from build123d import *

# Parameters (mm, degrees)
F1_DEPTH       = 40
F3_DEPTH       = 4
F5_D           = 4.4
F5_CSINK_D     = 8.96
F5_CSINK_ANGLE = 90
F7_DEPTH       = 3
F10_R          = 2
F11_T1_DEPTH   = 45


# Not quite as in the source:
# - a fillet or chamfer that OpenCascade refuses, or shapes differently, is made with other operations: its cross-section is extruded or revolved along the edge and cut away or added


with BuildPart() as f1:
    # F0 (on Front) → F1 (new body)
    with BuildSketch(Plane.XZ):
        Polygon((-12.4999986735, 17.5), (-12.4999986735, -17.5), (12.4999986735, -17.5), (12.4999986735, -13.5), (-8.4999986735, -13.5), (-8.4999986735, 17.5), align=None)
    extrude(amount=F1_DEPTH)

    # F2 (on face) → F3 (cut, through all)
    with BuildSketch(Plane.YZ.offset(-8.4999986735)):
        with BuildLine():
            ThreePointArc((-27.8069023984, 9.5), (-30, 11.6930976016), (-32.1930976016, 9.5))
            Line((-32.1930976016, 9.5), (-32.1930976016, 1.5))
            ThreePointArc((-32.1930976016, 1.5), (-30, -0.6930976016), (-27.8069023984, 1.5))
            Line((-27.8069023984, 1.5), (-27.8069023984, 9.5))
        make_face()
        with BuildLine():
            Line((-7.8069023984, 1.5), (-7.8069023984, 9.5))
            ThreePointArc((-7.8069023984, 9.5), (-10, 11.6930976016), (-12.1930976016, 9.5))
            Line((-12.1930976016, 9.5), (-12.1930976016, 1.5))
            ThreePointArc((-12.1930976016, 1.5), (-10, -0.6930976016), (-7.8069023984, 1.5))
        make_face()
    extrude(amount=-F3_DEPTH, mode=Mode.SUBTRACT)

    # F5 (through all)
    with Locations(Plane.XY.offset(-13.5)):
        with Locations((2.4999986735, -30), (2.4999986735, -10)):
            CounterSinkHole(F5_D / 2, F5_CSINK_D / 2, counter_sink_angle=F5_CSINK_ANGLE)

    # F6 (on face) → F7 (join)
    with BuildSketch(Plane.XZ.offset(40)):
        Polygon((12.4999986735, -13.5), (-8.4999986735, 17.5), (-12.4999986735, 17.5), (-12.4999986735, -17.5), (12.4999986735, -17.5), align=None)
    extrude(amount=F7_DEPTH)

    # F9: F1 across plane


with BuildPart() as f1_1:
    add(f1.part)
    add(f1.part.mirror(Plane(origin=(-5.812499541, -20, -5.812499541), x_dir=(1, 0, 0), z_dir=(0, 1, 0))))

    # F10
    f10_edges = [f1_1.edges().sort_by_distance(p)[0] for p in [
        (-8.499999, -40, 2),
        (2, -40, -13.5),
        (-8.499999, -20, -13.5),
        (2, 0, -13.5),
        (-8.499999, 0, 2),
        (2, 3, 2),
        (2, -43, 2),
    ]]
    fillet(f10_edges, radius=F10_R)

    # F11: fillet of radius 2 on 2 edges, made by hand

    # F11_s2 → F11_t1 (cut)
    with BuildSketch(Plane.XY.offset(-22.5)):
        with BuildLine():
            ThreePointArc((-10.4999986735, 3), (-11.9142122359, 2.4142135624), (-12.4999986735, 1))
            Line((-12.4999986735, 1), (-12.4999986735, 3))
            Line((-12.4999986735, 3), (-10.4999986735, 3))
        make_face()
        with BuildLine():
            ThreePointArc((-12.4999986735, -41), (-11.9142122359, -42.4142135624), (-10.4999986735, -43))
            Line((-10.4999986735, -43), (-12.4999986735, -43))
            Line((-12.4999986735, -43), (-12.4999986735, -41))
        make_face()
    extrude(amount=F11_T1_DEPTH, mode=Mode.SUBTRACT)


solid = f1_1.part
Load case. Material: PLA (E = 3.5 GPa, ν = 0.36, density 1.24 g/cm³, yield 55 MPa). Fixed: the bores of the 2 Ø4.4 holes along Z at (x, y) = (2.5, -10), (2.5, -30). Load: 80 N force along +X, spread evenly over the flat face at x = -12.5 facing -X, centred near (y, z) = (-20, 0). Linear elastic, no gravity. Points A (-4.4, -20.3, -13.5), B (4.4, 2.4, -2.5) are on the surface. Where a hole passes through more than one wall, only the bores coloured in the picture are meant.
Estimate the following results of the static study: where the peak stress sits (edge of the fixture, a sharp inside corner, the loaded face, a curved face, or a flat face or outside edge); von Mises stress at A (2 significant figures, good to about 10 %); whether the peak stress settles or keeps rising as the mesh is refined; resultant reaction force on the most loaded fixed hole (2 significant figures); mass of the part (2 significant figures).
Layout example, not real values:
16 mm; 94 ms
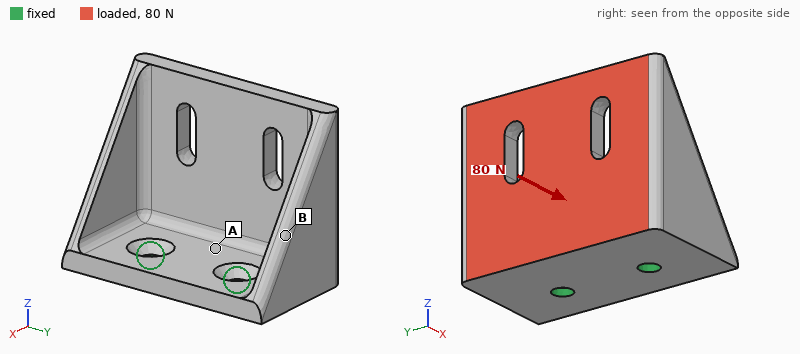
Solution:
edge of the fixture; 6.0 MPa; keeps rising; 43 N; 14 g
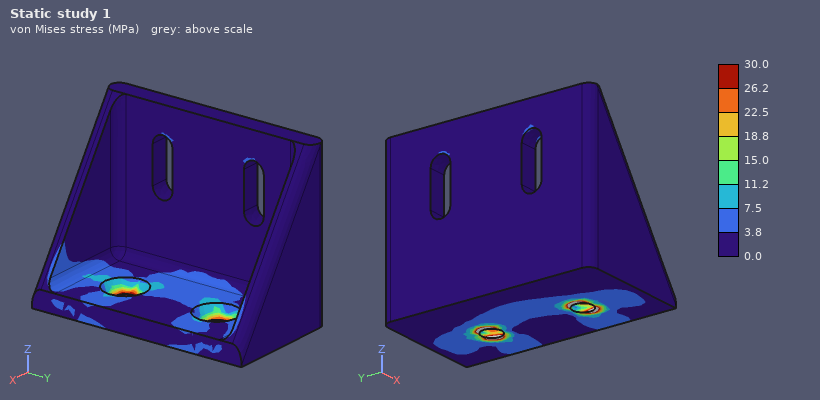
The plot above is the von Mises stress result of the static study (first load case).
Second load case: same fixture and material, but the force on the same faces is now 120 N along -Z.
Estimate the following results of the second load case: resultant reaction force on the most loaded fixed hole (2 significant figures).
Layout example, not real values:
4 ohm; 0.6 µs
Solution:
61 N
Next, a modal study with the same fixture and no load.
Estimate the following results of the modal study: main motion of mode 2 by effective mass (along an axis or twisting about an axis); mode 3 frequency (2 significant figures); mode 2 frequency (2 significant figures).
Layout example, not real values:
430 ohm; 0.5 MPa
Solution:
along Y; 2300 Hz; 1000 Hz
